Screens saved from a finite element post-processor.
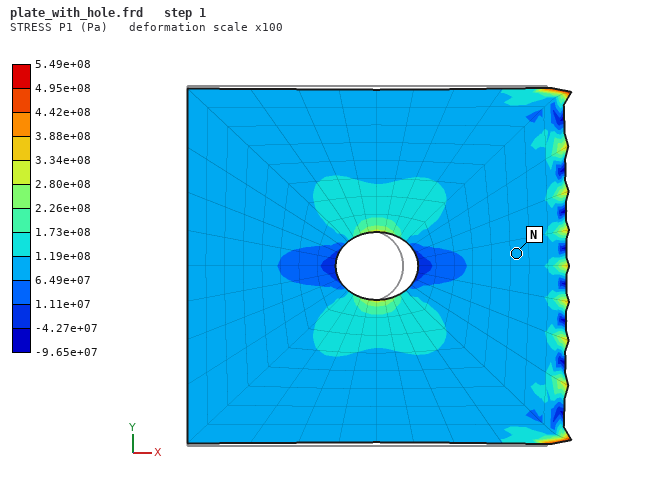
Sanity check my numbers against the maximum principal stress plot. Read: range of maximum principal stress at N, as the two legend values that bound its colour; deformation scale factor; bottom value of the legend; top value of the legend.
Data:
6.49e+07 to 1.19e+08 Pa
100
-9.65e+07 Pa
5.49e+08 Pa
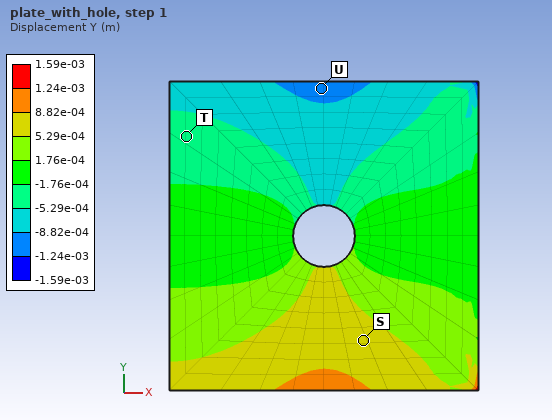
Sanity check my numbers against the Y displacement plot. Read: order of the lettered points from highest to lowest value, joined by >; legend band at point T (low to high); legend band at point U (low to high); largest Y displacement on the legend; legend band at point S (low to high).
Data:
S > T > U
-5.29e-04 to -1.76e-04 m
-1.24e-03 to -8.82e-04 m
1.59e-03 m
5.29e-04 to 8.82e-04 m
